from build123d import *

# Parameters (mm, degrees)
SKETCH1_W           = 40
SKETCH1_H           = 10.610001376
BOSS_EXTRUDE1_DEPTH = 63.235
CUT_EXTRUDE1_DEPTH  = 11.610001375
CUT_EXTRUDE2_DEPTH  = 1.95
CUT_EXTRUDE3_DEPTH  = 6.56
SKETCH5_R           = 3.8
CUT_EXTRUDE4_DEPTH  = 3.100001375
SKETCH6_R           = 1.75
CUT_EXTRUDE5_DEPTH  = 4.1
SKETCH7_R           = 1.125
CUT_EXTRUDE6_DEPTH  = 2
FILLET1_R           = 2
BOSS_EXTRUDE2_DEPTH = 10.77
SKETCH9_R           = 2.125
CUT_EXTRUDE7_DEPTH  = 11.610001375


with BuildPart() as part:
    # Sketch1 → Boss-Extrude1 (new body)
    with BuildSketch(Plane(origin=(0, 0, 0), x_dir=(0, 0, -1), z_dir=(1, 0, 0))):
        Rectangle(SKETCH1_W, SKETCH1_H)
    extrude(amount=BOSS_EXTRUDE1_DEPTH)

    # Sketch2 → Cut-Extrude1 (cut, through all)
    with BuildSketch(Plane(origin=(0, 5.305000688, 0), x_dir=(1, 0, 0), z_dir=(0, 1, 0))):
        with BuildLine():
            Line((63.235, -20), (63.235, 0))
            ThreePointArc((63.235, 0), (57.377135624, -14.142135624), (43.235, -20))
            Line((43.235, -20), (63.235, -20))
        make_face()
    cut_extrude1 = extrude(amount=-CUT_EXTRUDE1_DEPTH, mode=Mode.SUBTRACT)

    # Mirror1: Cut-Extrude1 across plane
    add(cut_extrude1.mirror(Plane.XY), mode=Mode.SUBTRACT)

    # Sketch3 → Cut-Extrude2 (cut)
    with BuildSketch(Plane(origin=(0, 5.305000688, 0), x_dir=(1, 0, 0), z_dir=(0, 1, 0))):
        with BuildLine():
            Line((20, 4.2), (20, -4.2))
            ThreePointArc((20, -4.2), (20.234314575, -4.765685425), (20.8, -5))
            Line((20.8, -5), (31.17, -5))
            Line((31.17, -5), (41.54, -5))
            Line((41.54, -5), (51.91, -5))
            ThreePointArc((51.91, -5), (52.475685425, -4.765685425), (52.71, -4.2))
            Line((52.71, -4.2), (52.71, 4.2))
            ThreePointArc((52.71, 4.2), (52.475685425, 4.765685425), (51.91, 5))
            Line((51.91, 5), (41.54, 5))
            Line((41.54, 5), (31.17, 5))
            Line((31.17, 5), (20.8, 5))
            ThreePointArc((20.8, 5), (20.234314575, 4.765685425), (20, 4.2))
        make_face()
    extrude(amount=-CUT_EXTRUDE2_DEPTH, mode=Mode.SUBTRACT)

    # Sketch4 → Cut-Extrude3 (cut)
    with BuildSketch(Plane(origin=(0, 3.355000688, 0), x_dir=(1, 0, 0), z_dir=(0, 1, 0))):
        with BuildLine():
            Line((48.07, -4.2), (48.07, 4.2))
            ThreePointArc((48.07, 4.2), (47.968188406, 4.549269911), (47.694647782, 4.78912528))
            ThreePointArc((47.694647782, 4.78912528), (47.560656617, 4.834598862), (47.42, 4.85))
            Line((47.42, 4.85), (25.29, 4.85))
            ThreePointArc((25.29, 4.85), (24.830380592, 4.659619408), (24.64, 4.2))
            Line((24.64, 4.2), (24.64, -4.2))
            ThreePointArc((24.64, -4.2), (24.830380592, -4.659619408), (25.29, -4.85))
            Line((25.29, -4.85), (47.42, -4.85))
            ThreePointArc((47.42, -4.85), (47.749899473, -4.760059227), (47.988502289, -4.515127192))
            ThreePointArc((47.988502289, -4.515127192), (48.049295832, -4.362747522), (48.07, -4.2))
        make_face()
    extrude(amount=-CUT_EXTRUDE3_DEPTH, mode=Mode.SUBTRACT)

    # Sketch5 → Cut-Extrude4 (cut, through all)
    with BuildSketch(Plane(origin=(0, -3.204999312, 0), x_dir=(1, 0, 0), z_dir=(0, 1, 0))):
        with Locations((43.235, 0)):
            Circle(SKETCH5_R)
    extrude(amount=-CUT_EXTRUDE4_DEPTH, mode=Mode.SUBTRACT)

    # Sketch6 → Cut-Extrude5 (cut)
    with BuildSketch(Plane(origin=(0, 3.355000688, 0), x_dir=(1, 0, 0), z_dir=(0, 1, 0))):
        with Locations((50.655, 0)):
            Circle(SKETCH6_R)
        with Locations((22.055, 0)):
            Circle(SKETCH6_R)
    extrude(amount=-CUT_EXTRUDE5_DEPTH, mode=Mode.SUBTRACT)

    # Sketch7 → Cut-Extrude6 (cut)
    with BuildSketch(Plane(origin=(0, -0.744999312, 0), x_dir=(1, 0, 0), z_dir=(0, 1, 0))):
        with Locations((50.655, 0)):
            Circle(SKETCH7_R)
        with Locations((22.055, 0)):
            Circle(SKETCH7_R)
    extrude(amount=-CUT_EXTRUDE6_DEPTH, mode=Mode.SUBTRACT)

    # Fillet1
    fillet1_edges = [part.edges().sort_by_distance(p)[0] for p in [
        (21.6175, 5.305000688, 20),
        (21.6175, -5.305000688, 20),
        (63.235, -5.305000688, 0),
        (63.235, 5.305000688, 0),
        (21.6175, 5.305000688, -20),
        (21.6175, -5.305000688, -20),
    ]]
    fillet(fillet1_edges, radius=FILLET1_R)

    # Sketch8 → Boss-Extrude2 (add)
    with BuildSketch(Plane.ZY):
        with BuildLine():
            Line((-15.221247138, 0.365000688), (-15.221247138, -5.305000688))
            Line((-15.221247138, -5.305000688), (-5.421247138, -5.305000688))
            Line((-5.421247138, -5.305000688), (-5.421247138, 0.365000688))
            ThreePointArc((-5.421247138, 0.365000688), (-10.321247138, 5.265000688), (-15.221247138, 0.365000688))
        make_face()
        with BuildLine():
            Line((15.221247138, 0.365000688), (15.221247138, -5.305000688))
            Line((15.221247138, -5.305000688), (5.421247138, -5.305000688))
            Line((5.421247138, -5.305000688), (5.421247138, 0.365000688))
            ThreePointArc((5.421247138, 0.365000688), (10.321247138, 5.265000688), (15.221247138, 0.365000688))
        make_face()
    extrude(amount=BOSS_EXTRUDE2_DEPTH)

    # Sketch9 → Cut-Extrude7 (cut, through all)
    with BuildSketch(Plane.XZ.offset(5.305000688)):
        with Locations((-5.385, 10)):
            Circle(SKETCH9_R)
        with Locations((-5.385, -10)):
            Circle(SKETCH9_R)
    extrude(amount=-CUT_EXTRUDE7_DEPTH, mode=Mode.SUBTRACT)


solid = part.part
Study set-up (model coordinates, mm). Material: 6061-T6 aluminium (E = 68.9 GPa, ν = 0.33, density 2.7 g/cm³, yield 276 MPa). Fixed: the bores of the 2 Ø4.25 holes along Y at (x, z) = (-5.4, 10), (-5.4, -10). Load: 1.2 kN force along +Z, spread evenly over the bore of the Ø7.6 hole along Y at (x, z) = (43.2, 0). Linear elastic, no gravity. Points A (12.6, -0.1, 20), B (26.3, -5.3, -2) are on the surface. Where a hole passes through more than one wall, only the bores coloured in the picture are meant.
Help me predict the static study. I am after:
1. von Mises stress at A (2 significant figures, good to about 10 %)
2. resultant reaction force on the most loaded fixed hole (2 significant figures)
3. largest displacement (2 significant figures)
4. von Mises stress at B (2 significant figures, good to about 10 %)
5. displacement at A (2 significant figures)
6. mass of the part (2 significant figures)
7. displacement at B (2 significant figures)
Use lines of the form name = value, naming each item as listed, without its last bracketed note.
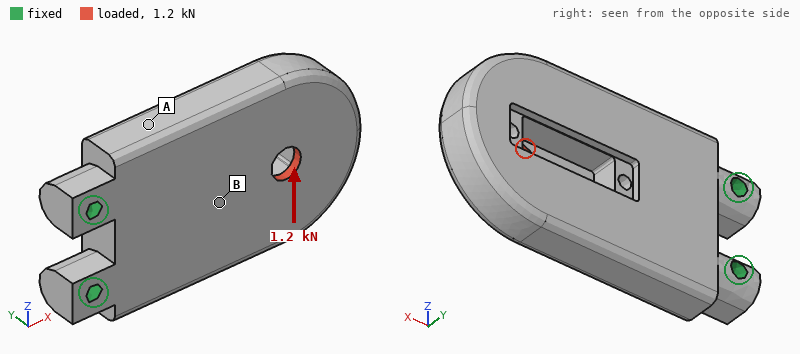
von Mises stress at A = 12 MPa
resultant reaction force on the most loaded fixed hole = 2.5 kN
largest displacement = 50 µm
von Mises stress at B = 23 MPa
displacement at A = 16 µm
mass of the part = 65 g
displacement at B = 22 µm
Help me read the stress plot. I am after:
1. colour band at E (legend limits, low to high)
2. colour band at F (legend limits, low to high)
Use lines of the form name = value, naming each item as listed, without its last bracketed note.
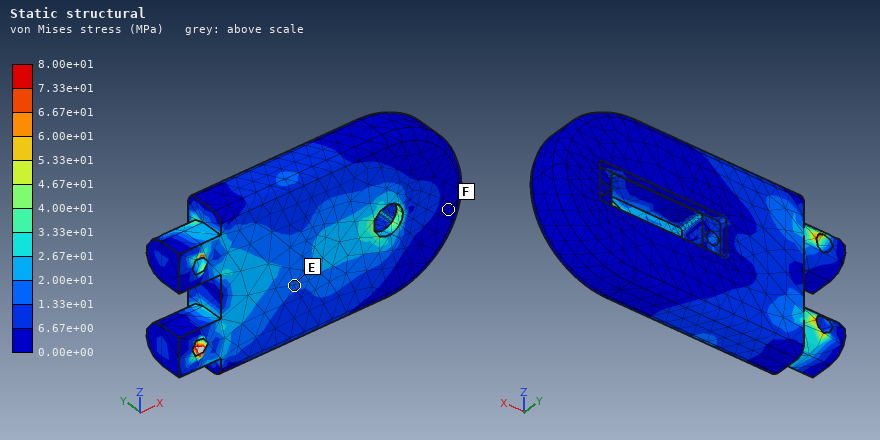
colour band at E = 1.33e+01 to 2.00e+01 MPa
colour band at F = 0.00e+00 to 6.67e+00 MPa
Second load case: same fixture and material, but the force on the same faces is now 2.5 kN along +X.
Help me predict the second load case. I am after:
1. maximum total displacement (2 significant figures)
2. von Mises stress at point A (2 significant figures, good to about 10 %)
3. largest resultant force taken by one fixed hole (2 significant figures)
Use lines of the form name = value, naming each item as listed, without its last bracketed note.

maximum total displacement = 0.11 mm
von Mises stress at point A = 6.0 MPa
largest resultant force taken by one fixed hole = 1.3 kN
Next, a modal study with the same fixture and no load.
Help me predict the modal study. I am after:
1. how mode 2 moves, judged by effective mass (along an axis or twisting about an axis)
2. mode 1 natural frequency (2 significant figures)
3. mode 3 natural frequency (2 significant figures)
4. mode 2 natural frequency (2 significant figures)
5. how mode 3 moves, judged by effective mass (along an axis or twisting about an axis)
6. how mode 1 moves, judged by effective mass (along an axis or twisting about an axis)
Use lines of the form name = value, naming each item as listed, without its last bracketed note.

how mode 2 moves, judged by effective mass = along Z
mode 1 natural frequency = 1700 Hz
mode 3 natural frequency = 5900 Hz
mode 2 natural frequency = 4700 Hz
how mode 3 moves, judged by effective mass = twisting about X
how mode 1 moves, judged by effective mass = along Y
